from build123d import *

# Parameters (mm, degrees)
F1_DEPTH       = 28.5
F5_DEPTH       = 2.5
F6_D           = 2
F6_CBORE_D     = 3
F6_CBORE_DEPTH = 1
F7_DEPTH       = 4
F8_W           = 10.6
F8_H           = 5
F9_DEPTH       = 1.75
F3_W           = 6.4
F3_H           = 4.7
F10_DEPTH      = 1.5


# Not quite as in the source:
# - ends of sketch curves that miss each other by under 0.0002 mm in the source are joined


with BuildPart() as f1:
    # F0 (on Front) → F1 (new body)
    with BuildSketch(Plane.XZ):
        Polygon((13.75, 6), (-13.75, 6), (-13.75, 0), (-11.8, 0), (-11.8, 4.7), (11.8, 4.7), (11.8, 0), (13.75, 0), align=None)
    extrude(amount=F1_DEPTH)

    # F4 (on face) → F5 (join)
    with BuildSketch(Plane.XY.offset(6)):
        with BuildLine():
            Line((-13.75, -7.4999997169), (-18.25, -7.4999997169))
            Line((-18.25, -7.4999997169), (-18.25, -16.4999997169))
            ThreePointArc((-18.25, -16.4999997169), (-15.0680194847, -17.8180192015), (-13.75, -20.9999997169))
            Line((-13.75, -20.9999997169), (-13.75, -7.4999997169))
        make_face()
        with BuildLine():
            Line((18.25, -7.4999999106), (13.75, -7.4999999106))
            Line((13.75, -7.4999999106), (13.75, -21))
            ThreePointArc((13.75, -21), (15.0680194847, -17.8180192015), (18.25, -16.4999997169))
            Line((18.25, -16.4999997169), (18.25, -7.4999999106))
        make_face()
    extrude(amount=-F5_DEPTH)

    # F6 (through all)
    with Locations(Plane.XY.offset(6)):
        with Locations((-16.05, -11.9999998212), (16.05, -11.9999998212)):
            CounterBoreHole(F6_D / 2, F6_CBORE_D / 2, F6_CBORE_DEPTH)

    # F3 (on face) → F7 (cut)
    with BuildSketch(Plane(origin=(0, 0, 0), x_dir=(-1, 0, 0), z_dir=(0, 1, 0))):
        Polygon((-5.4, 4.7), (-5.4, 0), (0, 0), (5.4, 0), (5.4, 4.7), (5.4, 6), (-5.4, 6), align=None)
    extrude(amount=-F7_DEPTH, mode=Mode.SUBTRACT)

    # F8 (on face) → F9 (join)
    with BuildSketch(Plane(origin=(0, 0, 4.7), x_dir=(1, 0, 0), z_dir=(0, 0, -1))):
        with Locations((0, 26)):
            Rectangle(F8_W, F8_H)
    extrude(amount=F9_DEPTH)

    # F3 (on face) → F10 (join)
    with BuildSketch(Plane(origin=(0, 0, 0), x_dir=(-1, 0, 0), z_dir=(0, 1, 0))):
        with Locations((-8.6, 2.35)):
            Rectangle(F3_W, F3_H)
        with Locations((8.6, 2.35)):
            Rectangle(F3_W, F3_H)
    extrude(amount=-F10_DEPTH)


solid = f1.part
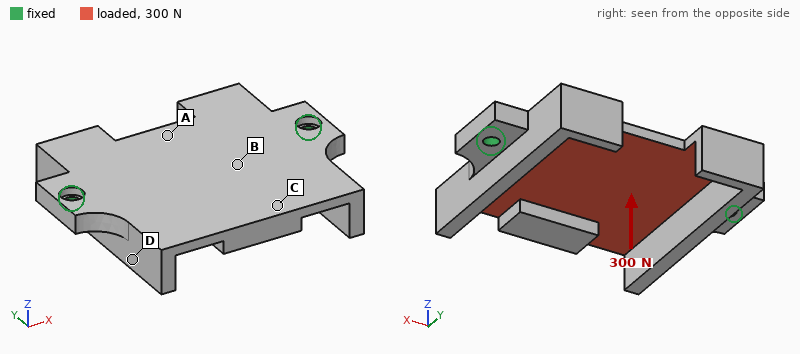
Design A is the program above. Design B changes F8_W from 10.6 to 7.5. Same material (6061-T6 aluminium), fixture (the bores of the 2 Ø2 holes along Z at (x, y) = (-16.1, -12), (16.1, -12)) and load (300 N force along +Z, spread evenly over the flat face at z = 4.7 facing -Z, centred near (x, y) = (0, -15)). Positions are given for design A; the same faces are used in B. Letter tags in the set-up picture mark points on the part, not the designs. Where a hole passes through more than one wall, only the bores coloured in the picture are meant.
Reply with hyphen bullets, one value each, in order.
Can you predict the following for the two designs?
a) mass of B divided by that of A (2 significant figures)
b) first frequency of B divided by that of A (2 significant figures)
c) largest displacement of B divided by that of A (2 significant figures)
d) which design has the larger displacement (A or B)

- 0.99
- 1.0
- 1.2
- B
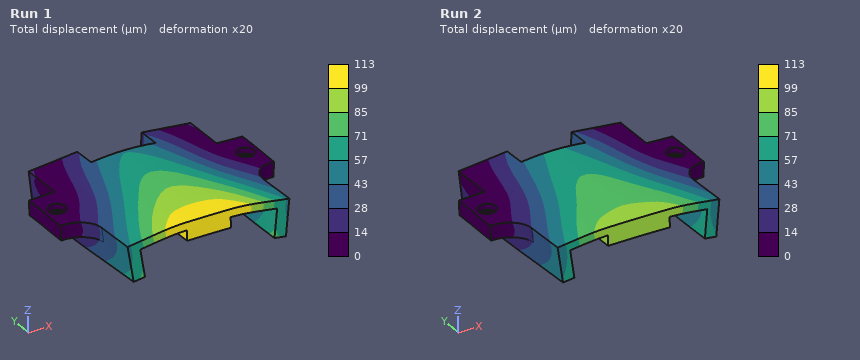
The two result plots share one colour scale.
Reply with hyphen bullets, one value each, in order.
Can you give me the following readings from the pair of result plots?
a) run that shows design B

- Run 1
